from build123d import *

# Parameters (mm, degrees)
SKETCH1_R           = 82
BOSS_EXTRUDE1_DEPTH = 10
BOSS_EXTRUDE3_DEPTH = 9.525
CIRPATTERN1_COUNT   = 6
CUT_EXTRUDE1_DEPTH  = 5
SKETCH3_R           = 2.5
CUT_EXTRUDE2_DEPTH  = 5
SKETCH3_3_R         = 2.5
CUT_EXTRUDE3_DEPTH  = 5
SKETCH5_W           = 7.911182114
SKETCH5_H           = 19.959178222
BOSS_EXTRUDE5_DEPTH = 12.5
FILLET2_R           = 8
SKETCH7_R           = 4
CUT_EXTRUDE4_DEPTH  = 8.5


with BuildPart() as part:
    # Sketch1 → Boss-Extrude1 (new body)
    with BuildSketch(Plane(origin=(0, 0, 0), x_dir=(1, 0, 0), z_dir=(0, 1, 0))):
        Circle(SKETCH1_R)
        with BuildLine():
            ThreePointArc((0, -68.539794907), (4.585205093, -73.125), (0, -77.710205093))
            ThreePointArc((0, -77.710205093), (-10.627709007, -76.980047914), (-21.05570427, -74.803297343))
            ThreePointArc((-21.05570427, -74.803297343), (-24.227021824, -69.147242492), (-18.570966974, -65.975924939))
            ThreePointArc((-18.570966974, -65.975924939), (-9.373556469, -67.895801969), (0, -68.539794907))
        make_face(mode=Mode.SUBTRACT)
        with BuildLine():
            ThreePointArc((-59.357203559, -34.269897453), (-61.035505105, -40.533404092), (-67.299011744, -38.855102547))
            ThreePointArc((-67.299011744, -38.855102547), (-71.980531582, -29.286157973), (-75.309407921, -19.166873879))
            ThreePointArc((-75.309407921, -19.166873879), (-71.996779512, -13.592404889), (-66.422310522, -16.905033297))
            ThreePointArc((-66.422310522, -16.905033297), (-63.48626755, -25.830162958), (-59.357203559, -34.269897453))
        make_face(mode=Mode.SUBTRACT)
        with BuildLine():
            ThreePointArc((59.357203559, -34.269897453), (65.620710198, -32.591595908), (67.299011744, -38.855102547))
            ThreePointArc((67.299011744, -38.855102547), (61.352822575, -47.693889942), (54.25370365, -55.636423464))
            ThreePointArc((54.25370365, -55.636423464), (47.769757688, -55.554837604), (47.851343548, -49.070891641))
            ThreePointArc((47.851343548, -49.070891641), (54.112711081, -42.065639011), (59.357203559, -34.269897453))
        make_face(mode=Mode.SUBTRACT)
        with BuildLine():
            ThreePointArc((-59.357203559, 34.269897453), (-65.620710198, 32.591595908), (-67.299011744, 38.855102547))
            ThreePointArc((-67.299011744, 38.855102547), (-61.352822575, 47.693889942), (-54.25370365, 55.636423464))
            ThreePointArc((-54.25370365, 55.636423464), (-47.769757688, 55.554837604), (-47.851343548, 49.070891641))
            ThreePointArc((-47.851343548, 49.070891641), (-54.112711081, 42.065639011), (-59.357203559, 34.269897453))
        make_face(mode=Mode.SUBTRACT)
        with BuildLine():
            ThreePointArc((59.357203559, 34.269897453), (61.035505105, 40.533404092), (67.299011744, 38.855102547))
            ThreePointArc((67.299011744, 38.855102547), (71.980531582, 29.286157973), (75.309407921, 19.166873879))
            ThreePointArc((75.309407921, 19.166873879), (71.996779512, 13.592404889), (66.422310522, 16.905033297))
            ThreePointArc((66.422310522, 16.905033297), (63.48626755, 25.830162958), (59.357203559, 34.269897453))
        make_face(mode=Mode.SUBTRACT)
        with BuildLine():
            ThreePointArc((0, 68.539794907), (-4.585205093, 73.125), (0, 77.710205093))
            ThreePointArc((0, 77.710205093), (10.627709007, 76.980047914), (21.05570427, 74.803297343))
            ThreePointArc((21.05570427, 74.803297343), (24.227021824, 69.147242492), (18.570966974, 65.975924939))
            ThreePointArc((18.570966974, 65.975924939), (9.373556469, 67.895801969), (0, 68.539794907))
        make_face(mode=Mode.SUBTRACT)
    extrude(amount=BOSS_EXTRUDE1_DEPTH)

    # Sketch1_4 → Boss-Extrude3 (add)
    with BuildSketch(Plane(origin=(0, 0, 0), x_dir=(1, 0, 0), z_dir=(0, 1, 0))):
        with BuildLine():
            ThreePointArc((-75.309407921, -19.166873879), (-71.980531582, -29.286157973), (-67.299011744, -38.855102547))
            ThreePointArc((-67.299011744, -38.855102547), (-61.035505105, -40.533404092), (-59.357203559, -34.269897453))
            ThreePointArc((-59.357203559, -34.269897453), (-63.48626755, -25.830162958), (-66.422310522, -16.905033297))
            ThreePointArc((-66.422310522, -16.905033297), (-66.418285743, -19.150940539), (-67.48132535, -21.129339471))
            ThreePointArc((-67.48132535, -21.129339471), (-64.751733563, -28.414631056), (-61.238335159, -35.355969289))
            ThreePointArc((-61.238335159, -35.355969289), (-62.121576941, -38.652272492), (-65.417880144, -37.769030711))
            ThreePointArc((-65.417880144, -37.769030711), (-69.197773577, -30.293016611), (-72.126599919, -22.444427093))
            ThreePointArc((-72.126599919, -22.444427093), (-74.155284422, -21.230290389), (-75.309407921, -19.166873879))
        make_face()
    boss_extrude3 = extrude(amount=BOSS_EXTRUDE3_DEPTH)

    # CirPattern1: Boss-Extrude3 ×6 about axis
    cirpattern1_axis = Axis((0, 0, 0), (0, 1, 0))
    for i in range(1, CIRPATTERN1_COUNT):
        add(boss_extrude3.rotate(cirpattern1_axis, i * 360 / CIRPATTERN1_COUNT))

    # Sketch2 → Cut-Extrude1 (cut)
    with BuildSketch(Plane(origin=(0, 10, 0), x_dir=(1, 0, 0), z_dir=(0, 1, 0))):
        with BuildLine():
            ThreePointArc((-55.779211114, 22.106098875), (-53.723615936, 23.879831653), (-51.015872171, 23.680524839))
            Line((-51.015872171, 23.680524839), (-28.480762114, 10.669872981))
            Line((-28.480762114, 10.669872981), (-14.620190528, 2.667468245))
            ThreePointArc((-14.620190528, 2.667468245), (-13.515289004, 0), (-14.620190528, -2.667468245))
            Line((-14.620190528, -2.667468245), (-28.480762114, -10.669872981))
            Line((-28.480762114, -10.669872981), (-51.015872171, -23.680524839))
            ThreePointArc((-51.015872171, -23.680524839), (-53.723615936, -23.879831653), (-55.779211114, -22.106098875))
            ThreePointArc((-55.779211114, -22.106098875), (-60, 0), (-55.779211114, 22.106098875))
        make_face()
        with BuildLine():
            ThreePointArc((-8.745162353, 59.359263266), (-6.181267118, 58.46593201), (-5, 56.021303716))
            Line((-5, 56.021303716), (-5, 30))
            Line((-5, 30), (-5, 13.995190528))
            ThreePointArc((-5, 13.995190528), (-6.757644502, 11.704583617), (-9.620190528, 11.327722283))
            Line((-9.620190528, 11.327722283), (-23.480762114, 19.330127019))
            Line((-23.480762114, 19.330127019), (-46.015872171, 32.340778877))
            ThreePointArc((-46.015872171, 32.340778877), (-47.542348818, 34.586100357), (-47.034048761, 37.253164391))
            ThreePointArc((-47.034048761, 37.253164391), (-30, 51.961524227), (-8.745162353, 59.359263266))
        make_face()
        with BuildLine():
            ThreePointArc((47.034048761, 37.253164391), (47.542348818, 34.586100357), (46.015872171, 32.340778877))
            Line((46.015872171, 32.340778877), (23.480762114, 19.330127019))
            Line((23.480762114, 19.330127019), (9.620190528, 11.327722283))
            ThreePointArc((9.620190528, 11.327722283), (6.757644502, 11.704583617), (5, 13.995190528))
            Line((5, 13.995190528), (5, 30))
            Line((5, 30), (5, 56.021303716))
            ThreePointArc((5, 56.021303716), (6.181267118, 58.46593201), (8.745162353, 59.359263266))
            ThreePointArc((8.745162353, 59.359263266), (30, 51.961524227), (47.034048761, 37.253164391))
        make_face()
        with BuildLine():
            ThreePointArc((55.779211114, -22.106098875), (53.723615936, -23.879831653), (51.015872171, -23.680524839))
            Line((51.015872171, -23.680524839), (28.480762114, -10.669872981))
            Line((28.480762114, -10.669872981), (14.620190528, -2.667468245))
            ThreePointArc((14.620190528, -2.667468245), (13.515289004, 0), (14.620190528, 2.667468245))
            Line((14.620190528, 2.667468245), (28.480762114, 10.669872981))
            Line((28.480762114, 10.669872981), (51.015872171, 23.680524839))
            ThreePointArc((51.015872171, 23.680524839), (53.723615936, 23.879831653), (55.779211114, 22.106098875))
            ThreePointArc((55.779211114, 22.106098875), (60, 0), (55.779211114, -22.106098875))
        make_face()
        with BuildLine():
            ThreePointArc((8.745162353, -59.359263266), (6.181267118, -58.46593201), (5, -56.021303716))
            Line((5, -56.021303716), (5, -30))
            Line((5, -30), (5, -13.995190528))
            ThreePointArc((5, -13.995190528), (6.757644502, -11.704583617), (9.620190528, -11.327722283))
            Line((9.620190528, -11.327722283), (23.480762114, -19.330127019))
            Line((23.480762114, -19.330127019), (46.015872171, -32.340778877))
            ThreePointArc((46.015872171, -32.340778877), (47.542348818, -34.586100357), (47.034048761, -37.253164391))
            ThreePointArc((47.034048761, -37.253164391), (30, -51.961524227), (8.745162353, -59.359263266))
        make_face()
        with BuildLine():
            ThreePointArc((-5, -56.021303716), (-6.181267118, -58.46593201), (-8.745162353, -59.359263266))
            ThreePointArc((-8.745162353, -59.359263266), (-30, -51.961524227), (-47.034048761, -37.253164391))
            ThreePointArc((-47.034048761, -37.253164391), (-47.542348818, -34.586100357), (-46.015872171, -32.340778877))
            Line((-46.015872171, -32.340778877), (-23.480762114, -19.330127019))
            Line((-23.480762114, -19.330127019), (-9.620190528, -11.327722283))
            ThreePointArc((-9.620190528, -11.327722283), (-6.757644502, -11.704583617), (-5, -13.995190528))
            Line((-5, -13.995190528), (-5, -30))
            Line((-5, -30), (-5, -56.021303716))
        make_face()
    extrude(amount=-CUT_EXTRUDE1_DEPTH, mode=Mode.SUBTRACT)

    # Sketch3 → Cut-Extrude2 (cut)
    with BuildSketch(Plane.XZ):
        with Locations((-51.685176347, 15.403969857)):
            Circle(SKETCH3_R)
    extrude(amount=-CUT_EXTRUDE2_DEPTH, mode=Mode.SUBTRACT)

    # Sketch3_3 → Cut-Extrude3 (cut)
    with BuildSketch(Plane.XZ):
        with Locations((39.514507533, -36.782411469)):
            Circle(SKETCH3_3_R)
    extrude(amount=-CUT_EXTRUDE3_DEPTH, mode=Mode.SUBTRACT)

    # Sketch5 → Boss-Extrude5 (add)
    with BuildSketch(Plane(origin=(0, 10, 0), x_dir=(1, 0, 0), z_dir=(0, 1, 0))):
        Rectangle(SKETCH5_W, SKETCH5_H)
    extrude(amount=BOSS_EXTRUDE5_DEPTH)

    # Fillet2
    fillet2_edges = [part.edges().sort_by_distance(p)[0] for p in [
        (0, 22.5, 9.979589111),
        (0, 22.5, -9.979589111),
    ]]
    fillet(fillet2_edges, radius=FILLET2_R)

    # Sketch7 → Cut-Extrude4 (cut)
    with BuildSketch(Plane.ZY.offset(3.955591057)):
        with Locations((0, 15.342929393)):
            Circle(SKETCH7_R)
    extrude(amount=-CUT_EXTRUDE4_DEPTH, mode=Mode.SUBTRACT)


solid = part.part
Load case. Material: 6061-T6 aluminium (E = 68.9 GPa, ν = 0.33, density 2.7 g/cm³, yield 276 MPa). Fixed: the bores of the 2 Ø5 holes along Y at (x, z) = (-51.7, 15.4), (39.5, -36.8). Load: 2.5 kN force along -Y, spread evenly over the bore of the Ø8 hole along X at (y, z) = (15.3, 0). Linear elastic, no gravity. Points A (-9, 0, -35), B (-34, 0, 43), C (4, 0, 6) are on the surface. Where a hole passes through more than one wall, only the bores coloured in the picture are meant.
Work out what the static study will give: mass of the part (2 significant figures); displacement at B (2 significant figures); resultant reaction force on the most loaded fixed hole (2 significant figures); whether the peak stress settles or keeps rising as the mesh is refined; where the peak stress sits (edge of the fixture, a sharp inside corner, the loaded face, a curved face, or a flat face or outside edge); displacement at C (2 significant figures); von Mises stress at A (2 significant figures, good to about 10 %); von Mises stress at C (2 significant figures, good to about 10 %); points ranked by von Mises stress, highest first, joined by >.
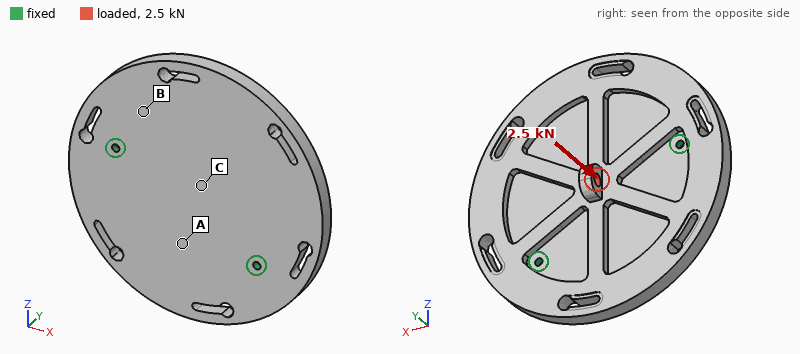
440 g
0.12 mm
1.4 kN
keeps rising
edge of the fixture
0.18 mm
19 MPa
35 MPa
C > A > B
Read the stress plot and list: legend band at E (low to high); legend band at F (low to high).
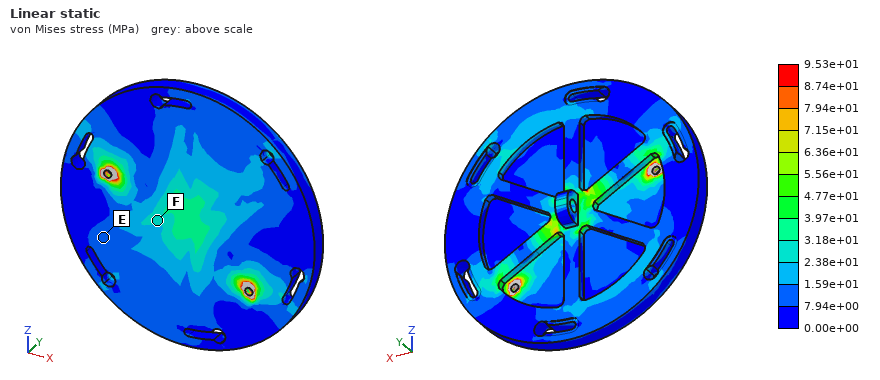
7.94e+00 to 1.59e+01 MPa
2.38e+01 to 3.18e+01 MPa
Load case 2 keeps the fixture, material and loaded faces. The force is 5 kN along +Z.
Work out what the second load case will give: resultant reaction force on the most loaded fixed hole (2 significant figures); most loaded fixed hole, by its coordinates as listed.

2.8 kN
(39.5, -36.8)
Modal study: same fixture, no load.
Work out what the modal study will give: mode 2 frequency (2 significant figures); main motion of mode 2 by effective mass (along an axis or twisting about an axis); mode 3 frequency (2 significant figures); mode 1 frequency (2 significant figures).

1200 Hz
along Y
1600 Hz
510 Hz
